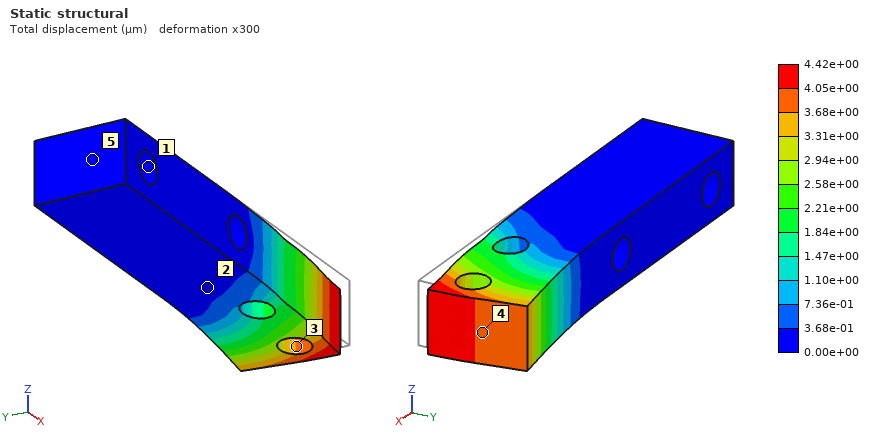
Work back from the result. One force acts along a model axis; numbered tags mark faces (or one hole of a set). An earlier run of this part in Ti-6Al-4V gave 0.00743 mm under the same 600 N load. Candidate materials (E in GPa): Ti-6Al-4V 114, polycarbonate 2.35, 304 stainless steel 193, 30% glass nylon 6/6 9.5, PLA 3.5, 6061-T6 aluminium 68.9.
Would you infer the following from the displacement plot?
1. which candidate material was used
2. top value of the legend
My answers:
304 stainless steel
4.42e+00 µm
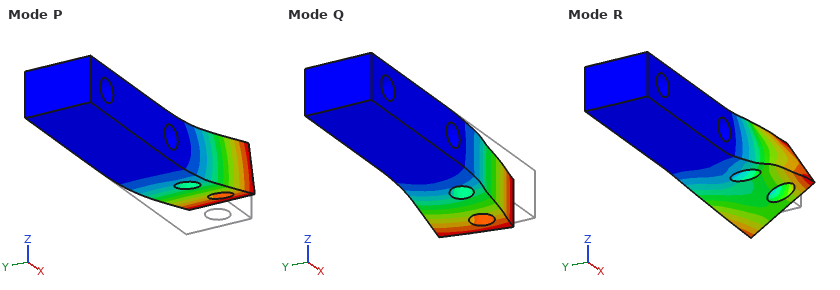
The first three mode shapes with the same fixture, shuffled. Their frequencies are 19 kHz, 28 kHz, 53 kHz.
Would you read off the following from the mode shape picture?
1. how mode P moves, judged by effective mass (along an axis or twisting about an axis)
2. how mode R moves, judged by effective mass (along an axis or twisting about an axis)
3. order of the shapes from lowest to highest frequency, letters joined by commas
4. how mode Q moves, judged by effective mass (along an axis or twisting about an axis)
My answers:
along Z
twisting about X
P, Q, R
along Y
